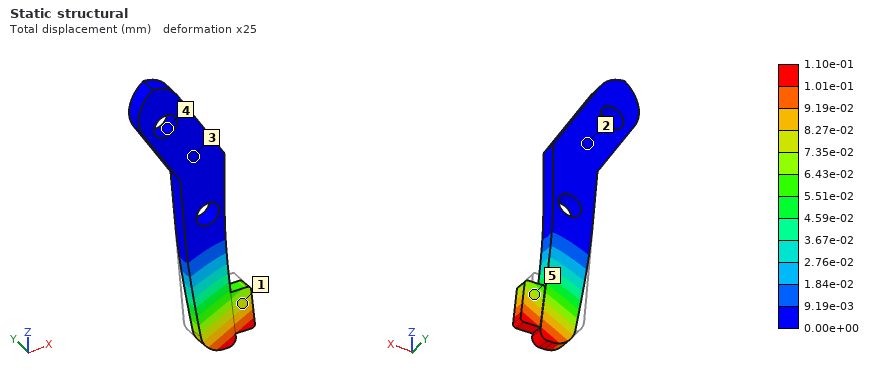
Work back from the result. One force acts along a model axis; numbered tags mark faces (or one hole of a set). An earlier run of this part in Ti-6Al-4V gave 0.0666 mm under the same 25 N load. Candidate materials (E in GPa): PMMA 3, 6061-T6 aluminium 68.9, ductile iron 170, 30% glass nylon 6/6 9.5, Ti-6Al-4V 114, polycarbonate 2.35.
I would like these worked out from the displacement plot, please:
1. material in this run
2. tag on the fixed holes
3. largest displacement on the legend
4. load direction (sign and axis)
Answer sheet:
6061-T6 aluminium
4
1.10e-01 mm
-Y
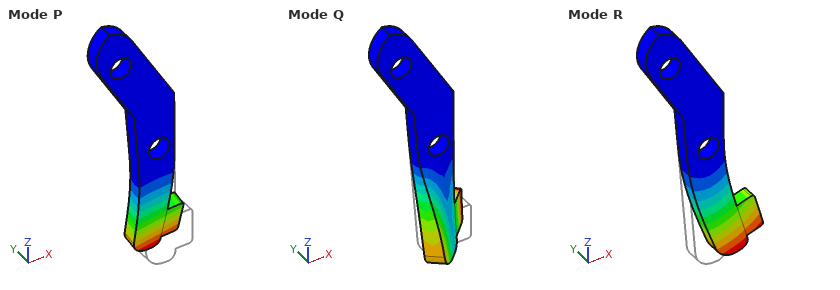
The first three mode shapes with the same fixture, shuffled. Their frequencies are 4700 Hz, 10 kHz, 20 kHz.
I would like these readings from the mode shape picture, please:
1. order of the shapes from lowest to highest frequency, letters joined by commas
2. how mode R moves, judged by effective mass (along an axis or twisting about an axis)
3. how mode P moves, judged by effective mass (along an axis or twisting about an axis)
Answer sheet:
P, R, Q
along X
along Y
